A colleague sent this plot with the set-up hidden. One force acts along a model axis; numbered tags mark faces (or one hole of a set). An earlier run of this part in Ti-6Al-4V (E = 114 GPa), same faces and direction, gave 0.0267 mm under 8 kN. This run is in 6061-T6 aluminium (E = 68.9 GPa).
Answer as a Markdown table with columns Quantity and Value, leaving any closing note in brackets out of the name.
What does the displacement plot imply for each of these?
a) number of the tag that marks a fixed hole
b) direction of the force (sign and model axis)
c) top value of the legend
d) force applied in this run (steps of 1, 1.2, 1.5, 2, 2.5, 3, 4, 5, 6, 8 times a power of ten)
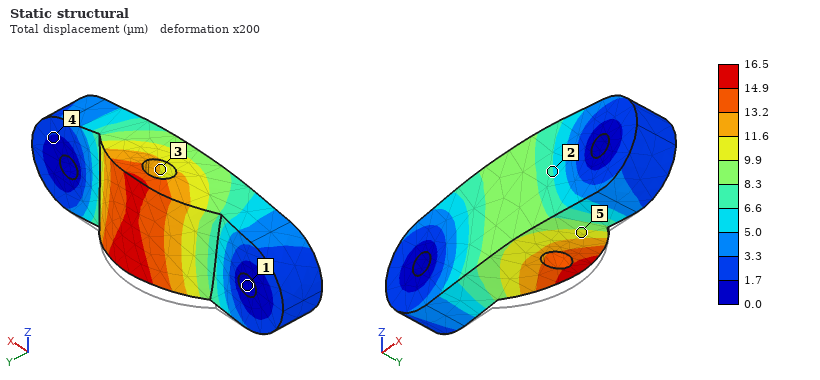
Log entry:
| Quantity | Value |
|---|---|
| number of the tag that marks a fixed hole | 1 |
| direction of the force | +Z |
| top value of the legend | 16.5 µm |
| force applied in this run | 3 kN |
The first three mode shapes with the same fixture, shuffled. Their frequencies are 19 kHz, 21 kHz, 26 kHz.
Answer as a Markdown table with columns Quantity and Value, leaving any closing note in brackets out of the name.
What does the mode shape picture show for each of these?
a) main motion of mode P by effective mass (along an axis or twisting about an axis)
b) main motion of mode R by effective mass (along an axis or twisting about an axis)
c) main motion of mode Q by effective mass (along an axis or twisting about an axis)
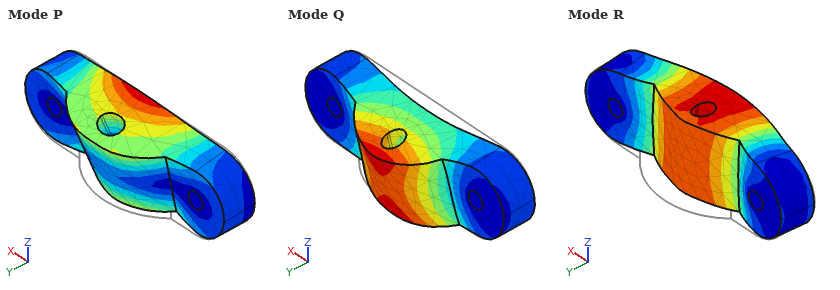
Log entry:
| Quantity | Value |
|---|---|
| main motion of mode P by effective mass | along Z |
| main motion of mode R by effective mass | along Y |
| main motion of mode Q by effective mass | along Z |
